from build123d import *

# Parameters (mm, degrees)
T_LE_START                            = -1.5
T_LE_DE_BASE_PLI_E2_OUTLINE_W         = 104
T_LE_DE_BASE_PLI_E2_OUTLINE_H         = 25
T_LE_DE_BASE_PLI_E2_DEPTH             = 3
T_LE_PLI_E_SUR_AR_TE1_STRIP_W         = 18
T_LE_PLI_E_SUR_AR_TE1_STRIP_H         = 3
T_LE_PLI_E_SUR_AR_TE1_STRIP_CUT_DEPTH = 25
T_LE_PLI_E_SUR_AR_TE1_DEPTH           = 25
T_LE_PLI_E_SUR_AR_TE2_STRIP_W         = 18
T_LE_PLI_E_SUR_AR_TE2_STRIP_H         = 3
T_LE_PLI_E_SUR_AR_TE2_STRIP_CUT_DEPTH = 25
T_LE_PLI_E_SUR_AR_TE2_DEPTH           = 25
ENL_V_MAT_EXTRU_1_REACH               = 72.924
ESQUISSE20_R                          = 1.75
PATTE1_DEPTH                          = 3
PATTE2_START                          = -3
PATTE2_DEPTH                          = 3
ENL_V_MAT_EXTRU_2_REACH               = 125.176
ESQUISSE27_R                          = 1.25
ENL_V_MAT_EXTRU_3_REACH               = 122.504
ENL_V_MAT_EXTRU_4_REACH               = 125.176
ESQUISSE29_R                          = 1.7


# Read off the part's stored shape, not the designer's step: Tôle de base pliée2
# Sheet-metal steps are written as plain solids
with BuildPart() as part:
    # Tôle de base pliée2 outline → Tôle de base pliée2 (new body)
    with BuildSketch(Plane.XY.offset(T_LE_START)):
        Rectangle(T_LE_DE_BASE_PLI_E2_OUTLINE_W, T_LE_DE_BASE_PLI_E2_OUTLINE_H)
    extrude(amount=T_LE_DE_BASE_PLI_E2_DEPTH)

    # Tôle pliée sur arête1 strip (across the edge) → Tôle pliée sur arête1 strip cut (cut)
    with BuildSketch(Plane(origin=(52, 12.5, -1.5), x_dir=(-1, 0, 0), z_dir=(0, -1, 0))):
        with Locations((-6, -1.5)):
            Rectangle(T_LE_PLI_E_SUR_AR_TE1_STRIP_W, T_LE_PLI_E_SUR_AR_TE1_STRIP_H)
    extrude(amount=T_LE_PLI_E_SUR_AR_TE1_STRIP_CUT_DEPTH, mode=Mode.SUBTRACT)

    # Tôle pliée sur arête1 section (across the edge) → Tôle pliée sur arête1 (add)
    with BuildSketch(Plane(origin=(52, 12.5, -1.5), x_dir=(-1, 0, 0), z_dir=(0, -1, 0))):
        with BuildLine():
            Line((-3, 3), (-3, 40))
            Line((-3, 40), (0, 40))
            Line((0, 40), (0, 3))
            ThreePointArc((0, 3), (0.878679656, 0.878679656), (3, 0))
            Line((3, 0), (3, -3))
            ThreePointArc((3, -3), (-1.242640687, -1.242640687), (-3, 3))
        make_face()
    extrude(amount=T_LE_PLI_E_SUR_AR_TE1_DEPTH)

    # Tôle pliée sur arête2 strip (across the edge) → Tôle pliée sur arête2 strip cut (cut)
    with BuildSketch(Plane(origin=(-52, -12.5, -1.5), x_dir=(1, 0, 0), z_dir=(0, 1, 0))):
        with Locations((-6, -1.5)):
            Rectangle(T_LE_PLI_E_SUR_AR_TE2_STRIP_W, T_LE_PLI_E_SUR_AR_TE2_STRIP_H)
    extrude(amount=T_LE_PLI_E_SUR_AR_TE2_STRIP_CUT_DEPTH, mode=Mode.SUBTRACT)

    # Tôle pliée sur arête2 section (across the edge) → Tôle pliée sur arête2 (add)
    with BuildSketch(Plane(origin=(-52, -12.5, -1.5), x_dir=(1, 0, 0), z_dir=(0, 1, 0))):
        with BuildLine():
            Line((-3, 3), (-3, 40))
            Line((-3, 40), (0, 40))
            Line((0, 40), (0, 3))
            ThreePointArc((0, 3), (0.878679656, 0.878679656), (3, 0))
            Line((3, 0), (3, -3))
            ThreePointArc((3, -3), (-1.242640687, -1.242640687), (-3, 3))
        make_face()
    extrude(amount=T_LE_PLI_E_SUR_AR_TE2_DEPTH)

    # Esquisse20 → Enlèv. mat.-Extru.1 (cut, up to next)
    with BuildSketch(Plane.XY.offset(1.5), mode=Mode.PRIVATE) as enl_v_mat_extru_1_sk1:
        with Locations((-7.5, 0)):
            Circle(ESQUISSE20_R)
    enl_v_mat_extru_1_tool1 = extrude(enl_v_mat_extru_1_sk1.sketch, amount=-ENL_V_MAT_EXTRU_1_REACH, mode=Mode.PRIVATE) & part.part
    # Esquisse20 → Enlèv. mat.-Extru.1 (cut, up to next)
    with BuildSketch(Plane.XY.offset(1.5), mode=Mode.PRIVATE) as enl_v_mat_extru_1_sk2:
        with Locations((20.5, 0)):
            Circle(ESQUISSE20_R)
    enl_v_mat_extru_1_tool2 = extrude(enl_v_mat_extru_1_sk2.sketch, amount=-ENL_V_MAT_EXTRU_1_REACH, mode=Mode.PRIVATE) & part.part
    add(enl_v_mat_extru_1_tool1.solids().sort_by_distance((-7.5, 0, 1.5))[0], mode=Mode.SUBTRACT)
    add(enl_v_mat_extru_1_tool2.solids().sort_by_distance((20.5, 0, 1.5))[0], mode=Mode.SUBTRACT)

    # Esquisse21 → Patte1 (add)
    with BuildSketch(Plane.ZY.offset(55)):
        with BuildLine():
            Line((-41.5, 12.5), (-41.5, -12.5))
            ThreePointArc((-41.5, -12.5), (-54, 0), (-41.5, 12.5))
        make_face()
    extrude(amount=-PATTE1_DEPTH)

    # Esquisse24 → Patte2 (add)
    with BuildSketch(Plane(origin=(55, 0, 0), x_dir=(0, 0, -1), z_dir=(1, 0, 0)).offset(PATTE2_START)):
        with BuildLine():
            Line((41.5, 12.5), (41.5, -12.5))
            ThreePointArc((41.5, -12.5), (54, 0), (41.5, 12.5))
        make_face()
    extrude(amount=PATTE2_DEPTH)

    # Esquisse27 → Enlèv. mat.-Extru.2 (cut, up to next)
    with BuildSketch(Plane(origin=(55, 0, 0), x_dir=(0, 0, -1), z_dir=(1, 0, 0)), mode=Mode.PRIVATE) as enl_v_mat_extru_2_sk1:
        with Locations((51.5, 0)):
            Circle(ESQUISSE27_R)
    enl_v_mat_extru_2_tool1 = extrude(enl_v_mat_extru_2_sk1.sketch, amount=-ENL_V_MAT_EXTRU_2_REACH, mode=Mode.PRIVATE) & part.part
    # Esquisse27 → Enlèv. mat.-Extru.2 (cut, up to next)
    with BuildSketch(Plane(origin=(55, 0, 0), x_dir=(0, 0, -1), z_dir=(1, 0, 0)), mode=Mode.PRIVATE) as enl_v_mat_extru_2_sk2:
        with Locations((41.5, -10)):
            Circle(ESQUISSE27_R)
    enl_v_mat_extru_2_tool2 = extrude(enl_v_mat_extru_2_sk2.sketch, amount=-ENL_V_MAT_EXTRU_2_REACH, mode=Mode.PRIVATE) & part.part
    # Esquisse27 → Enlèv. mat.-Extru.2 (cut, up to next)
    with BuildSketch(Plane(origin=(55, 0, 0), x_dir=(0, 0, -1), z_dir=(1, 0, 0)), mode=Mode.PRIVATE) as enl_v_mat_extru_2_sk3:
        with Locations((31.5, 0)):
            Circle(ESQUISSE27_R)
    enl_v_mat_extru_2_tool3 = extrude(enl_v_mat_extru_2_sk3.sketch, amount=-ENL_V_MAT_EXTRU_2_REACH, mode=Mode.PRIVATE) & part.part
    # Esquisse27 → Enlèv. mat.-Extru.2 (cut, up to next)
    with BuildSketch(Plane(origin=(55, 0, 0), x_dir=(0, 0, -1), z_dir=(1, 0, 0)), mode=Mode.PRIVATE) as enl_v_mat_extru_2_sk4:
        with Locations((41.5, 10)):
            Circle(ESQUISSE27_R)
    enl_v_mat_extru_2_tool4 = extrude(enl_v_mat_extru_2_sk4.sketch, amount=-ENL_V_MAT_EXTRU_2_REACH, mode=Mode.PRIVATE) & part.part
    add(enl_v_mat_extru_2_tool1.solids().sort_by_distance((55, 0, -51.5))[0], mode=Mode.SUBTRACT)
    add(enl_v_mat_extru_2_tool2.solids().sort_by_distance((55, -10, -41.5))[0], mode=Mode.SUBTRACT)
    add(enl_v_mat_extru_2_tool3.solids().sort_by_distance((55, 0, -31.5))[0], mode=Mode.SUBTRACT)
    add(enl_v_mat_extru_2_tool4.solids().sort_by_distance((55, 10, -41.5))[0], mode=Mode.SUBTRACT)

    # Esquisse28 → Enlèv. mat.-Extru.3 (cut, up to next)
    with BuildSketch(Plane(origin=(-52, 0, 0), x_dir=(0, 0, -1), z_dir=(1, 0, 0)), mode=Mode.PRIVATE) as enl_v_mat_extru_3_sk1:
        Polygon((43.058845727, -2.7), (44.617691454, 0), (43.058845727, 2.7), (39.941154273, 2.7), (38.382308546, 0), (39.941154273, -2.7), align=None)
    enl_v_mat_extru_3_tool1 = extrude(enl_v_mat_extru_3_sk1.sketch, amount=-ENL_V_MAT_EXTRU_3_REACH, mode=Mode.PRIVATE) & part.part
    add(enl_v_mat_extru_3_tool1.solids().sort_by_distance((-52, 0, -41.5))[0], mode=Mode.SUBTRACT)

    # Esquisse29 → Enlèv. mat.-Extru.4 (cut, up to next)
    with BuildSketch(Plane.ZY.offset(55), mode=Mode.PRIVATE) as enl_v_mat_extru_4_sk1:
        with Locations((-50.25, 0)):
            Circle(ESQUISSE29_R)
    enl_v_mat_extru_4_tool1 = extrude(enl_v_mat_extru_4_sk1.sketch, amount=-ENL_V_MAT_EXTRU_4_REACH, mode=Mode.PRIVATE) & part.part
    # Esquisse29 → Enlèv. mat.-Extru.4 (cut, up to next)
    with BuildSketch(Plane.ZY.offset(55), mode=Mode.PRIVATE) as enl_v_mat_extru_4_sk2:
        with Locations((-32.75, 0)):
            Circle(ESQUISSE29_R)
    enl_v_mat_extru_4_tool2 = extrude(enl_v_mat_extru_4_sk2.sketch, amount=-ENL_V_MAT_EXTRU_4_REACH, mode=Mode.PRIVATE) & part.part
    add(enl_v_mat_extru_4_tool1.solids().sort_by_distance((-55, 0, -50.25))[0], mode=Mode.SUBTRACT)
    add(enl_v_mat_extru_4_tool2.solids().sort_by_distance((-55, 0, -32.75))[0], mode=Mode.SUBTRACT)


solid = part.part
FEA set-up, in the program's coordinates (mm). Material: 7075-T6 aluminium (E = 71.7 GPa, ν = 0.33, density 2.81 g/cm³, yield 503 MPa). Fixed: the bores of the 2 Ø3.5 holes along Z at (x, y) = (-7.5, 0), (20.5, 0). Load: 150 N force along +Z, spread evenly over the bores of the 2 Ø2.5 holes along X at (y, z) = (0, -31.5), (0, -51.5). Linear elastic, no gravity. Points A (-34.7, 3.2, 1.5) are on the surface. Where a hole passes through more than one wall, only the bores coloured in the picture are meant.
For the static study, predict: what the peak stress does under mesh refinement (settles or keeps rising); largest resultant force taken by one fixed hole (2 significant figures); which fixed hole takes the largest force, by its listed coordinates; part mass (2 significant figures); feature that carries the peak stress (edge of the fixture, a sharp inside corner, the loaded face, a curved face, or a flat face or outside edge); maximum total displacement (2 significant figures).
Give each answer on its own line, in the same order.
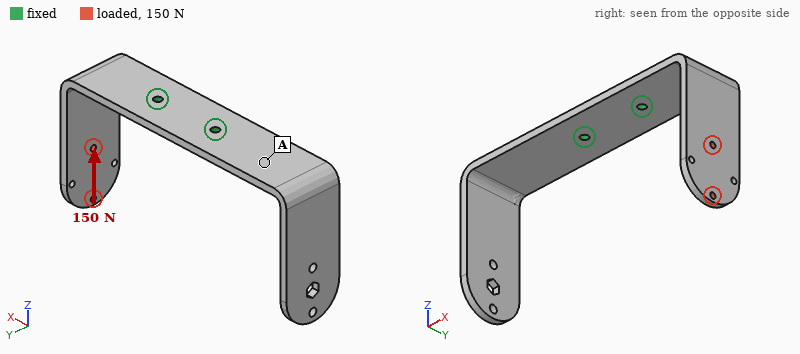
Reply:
keeps rising
190 N
(20.5, 0)
43 g
edge of the fixture
1.2 mm
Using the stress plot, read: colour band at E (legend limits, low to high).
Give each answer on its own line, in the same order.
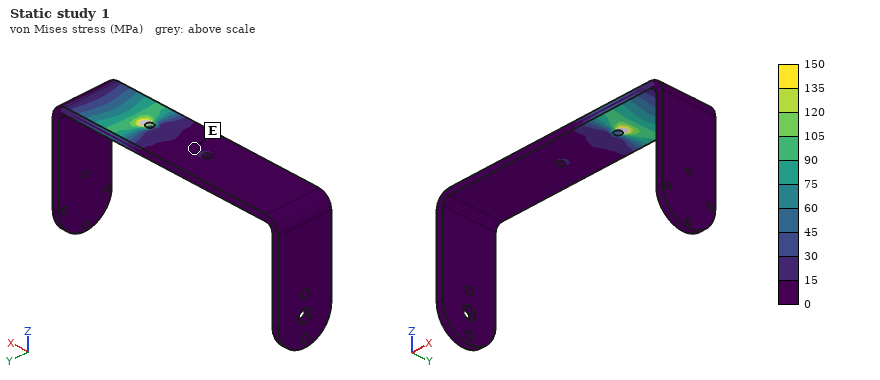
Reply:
0 to 15 MPa
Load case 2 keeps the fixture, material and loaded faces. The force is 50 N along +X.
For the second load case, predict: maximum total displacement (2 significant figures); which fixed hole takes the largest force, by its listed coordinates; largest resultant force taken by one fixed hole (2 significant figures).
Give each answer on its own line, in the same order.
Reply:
1.3 mm
(20.5, 0)
44 N
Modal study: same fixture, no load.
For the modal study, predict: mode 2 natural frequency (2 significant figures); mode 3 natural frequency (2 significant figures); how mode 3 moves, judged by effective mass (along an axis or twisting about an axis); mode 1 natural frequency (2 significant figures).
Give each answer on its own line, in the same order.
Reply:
460 Hz
580 Hz
along Y
360 Hz
